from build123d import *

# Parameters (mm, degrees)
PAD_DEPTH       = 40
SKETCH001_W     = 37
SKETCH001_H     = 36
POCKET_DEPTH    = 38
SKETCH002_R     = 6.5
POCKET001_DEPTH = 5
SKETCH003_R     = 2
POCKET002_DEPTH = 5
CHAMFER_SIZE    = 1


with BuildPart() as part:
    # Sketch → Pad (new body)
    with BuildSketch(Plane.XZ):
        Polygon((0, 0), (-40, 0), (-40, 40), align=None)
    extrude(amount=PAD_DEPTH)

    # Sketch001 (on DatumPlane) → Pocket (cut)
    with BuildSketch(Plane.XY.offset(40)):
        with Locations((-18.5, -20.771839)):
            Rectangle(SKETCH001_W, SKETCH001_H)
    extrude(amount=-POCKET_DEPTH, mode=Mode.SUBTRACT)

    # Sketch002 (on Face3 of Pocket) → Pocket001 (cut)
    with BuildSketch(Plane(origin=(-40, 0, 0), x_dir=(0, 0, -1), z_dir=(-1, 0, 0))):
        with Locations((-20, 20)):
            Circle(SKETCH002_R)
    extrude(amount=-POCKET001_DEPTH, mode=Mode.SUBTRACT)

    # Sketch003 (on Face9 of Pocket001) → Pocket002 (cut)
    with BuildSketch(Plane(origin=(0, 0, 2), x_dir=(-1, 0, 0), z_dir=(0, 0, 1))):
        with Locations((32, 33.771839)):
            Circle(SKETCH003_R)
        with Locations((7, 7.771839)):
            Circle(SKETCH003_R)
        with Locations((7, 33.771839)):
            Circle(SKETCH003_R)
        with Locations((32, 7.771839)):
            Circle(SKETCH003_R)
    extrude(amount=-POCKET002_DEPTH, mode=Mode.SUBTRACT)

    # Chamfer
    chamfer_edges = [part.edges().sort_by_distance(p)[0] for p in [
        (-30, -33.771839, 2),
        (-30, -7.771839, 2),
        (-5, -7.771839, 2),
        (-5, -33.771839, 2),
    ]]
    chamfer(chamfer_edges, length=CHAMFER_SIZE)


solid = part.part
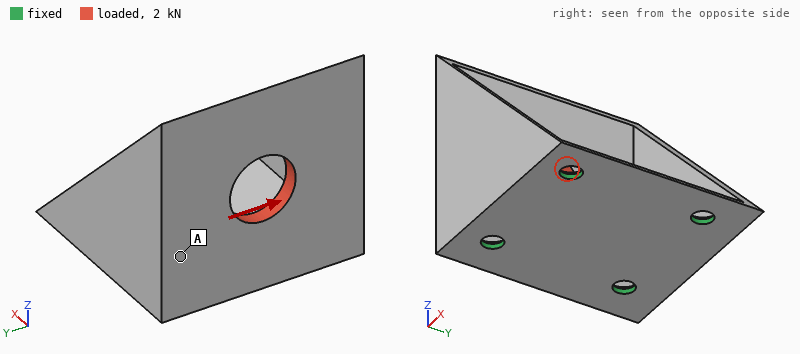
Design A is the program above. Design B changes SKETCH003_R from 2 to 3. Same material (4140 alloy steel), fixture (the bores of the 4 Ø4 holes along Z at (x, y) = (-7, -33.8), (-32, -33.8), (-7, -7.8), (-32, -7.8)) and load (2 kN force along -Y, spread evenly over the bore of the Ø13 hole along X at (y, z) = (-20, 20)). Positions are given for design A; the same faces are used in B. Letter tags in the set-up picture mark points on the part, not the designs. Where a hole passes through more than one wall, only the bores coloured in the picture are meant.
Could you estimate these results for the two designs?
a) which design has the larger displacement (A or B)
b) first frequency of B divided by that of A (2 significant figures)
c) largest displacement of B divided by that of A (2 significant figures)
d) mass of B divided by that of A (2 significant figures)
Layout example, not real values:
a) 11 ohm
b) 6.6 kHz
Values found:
a) A
b) 1.1
c) 0.64
d) 0.99
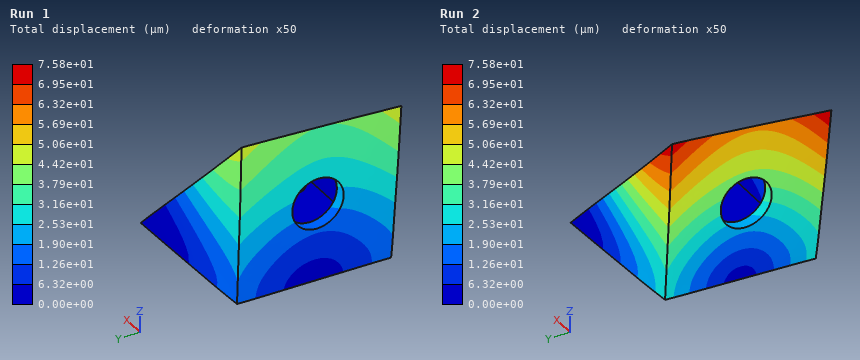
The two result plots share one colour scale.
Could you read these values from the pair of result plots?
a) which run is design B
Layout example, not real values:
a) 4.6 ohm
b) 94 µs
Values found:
a) Run 1
